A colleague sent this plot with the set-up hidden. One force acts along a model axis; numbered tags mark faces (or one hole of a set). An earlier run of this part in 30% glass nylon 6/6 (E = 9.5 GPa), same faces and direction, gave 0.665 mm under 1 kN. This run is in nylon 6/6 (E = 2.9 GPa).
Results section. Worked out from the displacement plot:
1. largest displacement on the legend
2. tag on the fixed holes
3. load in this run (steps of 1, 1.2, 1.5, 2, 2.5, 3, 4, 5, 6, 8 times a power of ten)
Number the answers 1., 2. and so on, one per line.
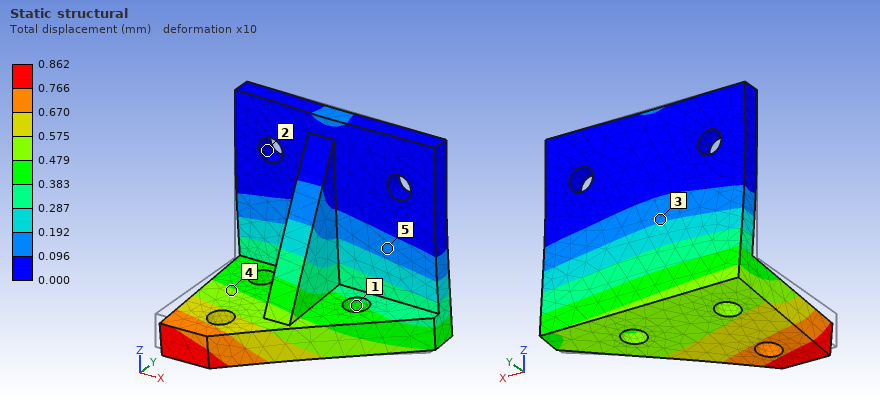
1. 0.862 mm
2. 2
3. 400 N
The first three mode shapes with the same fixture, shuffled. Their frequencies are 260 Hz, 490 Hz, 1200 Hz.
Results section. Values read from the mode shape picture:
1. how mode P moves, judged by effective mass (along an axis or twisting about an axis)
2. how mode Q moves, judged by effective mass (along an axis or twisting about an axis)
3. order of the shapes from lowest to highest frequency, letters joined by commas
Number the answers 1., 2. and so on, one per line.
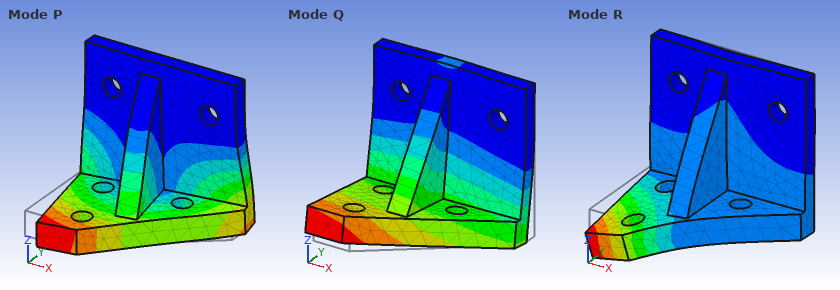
1. along X
2. along Y
3. Q, P, R
